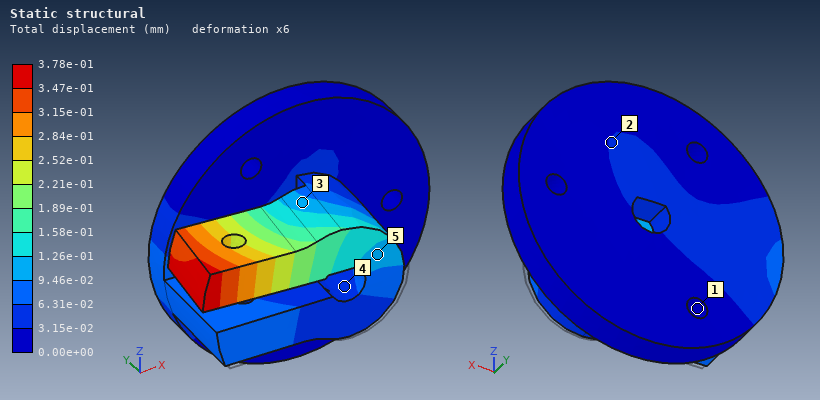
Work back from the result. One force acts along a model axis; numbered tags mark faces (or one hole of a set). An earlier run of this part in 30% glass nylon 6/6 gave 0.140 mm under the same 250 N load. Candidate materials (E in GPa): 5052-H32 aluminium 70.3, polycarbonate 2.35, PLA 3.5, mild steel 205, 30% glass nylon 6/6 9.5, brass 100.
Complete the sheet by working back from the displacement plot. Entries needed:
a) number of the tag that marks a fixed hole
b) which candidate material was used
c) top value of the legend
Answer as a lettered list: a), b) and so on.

a) 1
b) PLA
c) 3.78e-01 mm
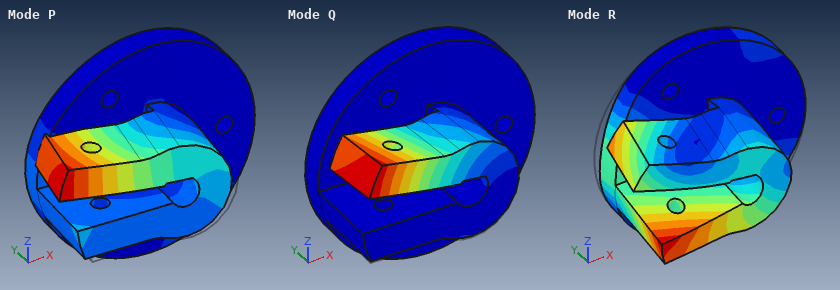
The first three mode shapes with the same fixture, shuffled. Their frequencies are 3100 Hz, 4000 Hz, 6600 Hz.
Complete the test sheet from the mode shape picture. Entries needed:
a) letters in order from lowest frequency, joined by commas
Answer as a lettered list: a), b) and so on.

a) Q, P, R
